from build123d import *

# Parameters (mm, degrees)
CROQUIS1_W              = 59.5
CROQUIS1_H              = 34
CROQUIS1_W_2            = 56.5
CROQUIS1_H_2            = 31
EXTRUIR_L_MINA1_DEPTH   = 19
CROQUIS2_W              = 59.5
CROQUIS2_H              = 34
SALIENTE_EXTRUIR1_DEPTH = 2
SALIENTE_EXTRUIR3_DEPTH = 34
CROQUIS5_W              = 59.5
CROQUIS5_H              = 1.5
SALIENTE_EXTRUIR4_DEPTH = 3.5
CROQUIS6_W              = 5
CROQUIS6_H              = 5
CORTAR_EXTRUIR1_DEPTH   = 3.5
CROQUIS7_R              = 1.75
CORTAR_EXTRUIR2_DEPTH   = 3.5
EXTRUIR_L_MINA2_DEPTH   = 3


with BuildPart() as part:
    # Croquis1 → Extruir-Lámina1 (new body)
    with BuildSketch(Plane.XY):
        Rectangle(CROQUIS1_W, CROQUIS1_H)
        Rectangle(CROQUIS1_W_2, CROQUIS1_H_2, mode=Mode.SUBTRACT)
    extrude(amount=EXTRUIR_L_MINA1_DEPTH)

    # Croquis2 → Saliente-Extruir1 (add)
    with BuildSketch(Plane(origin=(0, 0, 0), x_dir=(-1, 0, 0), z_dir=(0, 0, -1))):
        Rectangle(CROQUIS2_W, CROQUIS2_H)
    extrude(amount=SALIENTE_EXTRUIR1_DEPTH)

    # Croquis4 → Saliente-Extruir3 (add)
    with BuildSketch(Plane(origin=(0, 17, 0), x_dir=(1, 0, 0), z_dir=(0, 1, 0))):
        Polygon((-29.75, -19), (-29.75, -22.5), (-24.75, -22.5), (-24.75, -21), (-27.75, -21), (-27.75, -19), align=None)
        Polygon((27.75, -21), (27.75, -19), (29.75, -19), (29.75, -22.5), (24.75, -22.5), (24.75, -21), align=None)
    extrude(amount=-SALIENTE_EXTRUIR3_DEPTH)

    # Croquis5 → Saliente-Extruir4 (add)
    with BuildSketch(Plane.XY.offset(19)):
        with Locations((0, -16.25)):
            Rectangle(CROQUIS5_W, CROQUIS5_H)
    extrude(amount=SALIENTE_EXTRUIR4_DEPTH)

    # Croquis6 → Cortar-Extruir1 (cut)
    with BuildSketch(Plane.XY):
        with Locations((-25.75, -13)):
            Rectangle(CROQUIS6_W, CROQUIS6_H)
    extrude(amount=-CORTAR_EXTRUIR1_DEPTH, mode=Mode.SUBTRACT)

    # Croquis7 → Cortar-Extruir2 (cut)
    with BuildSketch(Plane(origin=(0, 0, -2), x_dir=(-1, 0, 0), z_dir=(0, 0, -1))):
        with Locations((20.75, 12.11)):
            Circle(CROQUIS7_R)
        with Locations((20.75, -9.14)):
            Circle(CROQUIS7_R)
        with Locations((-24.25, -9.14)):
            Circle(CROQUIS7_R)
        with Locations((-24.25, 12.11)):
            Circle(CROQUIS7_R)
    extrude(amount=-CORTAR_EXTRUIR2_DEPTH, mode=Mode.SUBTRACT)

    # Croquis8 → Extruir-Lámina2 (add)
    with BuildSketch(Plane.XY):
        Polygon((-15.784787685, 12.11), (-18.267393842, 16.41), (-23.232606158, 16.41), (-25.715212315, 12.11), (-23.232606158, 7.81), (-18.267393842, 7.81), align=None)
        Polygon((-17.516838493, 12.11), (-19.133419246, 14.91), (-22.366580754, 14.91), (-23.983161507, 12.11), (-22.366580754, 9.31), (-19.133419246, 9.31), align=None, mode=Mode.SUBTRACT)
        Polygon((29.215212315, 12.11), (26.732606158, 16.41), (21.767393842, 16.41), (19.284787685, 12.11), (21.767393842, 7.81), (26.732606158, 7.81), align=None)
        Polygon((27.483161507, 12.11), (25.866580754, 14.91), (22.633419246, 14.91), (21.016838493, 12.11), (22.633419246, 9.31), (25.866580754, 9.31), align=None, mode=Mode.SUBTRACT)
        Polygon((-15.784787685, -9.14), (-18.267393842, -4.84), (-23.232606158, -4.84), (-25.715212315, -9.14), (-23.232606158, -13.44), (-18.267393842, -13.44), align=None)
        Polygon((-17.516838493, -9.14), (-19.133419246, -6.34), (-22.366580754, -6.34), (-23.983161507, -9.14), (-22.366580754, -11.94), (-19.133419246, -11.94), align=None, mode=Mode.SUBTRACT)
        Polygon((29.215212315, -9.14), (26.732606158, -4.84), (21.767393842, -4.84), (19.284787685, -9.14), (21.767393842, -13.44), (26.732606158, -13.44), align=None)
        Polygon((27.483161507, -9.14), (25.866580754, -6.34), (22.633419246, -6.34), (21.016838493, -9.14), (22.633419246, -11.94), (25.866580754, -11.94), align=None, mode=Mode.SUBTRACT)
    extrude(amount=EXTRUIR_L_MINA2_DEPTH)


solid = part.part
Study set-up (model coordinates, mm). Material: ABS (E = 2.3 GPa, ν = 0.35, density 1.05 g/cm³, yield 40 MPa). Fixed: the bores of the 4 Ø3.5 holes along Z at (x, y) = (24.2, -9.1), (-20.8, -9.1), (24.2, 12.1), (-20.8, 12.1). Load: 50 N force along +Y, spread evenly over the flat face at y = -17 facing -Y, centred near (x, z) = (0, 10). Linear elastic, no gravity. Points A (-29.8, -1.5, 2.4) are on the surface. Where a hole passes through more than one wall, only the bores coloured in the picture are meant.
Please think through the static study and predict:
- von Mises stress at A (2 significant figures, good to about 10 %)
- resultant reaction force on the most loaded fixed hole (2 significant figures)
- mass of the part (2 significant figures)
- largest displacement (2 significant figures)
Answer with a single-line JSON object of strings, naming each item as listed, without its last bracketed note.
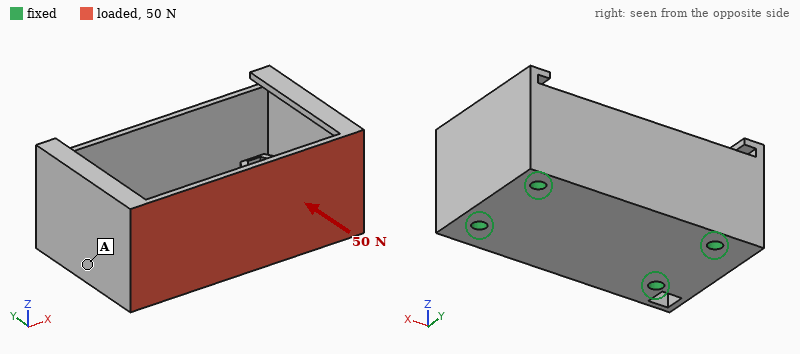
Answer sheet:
{"von Mises stress at A": "1.2 MPa", "resultant reaction force on the most loaded fixed hole": "18 N", "mass of the part": "11 g", "largest displacement": "0.84 mm"}
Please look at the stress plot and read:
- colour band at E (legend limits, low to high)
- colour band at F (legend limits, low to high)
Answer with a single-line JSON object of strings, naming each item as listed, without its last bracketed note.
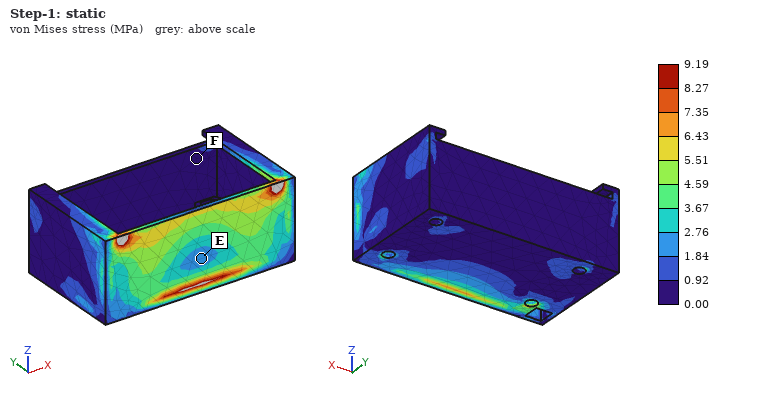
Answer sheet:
{"colour band at E": "1.84 to 2.76 MPa", "colour band at F": "0.00 to 0.92 MPa"}
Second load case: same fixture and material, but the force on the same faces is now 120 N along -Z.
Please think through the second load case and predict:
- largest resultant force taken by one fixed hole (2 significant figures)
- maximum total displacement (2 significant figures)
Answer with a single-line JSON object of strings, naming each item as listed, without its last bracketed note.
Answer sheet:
{"largest resultant force taken by one fixed hole": "78 N", "maximum total displacement": "0.35 mm"}
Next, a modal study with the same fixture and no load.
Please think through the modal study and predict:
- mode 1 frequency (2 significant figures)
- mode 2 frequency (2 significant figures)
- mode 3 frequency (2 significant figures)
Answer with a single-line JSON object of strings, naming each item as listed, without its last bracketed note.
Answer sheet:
{"mode 1 frequency": "1100 Hz", "mode 2 frequency": "1200 Hz", "mode 3 frequency": "2000 Hz"}
